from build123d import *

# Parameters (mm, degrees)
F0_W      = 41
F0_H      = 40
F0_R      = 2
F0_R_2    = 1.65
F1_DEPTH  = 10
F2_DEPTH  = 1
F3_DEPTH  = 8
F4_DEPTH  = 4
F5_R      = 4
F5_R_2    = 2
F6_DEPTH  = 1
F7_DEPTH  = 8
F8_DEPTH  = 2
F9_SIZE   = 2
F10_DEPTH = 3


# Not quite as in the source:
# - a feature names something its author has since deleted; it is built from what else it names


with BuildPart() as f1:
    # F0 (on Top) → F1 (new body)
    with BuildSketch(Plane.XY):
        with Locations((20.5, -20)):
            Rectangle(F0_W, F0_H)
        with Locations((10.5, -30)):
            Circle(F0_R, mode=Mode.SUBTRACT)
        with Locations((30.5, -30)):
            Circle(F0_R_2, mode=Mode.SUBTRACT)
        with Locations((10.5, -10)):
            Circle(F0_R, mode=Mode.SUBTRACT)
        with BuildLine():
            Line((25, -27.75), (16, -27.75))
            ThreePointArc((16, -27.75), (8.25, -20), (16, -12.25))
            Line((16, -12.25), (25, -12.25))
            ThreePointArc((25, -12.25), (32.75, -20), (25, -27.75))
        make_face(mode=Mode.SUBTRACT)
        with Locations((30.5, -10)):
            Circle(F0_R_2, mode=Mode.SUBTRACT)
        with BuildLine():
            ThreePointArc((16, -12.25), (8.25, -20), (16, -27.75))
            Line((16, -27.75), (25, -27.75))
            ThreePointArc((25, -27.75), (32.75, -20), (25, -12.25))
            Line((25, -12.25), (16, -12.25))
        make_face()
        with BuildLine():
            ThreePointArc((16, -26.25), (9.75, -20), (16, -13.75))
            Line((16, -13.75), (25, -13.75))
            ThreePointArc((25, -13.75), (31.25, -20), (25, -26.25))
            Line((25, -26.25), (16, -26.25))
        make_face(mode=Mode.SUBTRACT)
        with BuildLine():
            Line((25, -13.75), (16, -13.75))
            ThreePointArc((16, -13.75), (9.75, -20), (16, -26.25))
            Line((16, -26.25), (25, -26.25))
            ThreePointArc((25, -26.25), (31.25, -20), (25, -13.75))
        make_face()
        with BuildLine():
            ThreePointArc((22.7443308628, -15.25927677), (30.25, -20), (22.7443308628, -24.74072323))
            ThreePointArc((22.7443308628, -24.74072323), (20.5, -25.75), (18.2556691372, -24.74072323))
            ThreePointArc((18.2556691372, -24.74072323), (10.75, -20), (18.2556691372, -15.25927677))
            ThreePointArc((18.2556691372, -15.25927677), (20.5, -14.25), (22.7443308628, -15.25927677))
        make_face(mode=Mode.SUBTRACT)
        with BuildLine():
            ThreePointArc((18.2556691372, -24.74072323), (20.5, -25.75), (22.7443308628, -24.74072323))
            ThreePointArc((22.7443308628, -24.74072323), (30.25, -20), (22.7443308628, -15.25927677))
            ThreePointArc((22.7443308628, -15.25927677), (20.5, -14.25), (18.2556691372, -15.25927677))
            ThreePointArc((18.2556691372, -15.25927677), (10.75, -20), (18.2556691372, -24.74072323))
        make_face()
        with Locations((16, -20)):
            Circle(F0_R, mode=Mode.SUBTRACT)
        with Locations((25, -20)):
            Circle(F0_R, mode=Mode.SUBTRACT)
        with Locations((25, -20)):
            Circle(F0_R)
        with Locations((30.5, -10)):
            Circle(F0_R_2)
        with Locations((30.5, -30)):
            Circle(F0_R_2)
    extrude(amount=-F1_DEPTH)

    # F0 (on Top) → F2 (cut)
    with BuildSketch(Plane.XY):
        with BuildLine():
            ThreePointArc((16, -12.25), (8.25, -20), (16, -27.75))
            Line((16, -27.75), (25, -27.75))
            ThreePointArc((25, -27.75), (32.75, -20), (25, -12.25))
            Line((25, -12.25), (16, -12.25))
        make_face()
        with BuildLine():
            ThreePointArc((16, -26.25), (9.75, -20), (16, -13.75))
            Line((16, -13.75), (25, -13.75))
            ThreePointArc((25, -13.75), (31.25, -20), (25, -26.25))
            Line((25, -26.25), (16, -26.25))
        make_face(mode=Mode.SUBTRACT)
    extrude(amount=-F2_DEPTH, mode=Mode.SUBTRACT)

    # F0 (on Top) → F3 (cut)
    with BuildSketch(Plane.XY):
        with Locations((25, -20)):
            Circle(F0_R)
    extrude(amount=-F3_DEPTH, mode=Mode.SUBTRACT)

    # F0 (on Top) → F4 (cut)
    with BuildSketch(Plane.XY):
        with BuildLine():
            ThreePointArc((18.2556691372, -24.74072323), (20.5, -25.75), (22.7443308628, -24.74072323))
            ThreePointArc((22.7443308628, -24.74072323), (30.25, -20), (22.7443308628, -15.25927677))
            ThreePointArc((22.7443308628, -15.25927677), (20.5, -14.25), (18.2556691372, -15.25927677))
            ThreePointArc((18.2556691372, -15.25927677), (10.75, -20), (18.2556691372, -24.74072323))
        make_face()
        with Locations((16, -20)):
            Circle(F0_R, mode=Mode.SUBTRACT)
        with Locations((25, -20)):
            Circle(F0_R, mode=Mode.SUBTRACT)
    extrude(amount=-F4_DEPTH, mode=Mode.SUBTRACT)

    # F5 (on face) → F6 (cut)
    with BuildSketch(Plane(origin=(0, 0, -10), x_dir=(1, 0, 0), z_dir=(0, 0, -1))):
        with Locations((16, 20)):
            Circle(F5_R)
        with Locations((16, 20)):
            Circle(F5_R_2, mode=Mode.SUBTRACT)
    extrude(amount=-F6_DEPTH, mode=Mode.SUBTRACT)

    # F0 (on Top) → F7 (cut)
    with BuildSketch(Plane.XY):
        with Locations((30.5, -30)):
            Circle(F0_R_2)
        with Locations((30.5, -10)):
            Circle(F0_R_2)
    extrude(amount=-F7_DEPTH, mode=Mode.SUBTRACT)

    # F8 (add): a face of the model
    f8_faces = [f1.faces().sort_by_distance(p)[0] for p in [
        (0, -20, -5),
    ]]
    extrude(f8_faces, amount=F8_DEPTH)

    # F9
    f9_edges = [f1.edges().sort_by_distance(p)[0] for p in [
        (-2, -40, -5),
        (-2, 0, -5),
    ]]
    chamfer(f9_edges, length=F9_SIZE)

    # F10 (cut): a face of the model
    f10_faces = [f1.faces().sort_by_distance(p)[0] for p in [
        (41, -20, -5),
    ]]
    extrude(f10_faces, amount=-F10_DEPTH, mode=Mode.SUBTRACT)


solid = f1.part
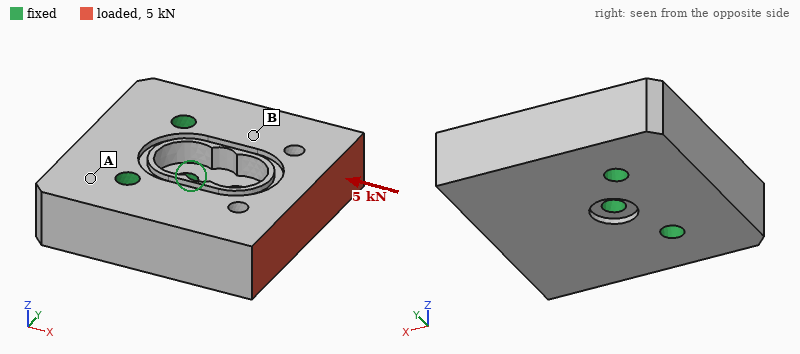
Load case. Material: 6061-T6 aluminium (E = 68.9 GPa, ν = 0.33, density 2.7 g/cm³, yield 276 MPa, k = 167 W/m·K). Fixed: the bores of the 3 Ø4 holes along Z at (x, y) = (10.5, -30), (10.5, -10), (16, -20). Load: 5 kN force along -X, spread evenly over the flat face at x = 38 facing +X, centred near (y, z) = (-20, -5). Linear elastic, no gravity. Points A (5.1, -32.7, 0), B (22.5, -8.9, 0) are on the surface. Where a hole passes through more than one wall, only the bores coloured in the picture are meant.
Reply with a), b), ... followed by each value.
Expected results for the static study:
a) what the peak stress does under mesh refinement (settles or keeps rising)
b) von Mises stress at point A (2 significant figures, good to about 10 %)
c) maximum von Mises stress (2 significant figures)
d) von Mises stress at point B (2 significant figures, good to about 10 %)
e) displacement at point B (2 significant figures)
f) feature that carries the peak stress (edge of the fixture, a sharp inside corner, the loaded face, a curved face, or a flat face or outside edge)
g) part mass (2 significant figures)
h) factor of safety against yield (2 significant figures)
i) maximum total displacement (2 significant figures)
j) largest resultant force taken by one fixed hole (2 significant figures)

a) settles
b) 6.7 MPa
c) 62 MPa
d) 18 MPa
e) 3.8 µm
f) a curved face
g) 39 g
h) 4.4
i) 10 µm
j) 2.0 kN
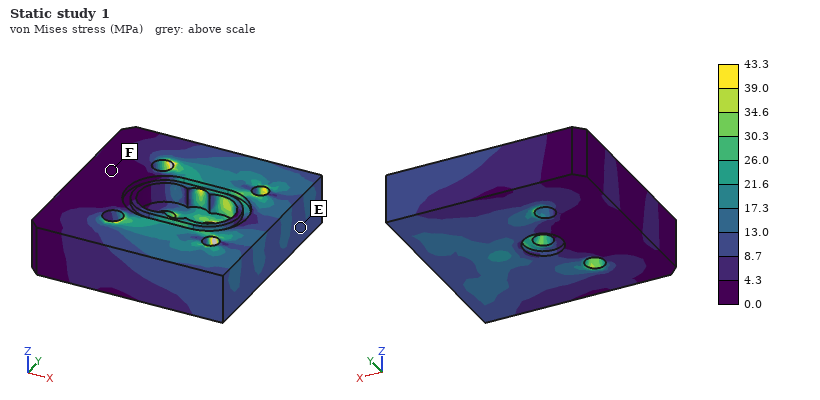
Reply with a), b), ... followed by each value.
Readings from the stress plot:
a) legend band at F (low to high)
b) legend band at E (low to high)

a) 0.0 to 4.3 MPa
b) 8.7 to 13.0 MPa
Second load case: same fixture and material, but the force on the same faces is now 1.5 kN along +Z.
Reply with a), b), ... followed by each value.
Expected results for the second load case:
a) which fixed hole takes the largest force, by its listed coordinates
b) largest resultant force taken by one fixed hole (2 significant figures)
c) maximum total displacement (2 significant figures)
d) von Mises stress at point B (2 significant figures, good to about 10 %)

a) (16, -20)
b) 1.4 kN
c) 59 µm
d) 44 MPa
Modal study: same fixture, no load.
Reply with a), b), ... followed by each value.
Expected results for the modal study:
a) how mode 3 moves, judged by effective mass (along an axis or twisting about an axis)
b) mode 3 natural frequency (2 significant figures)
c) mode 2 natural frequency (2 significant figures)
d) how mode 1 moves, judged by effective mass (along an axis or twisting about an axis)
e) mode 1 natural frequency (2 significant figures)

a) along Y
b) 19 kHz
c) 14 kHz
d) along Z
e) 9700 Hz
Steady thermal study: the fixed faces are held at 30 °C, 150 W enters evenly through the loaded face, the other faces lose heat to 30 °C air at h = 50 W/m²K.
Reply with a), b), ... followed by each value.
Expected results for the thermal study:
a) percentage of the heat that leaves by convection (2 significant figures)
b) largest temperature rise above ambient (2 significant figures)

a) 3.6 %
b) 66 K
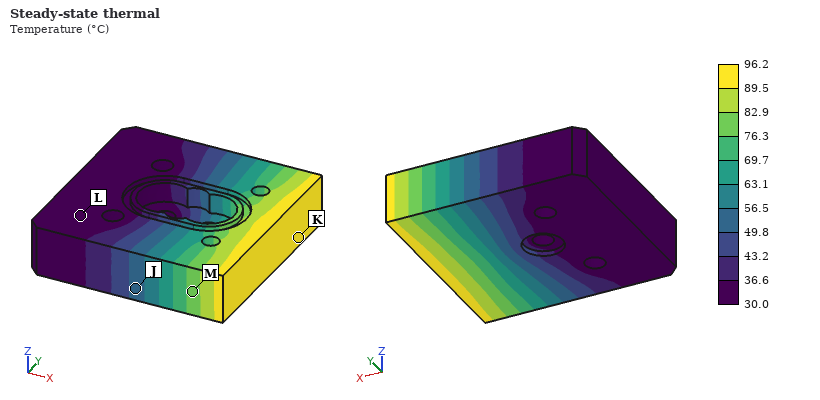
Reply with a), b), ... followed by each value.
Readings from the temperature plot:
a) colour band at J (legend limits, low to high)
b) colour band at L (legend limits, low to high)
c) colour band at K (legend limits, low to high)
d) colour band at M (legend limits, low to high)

a) 49.8 to 56.5 °C
b) 30.0 to 36.6 °C
c) 89.5 to 96.2 °C
d) 76.3 to 82.9 °C
